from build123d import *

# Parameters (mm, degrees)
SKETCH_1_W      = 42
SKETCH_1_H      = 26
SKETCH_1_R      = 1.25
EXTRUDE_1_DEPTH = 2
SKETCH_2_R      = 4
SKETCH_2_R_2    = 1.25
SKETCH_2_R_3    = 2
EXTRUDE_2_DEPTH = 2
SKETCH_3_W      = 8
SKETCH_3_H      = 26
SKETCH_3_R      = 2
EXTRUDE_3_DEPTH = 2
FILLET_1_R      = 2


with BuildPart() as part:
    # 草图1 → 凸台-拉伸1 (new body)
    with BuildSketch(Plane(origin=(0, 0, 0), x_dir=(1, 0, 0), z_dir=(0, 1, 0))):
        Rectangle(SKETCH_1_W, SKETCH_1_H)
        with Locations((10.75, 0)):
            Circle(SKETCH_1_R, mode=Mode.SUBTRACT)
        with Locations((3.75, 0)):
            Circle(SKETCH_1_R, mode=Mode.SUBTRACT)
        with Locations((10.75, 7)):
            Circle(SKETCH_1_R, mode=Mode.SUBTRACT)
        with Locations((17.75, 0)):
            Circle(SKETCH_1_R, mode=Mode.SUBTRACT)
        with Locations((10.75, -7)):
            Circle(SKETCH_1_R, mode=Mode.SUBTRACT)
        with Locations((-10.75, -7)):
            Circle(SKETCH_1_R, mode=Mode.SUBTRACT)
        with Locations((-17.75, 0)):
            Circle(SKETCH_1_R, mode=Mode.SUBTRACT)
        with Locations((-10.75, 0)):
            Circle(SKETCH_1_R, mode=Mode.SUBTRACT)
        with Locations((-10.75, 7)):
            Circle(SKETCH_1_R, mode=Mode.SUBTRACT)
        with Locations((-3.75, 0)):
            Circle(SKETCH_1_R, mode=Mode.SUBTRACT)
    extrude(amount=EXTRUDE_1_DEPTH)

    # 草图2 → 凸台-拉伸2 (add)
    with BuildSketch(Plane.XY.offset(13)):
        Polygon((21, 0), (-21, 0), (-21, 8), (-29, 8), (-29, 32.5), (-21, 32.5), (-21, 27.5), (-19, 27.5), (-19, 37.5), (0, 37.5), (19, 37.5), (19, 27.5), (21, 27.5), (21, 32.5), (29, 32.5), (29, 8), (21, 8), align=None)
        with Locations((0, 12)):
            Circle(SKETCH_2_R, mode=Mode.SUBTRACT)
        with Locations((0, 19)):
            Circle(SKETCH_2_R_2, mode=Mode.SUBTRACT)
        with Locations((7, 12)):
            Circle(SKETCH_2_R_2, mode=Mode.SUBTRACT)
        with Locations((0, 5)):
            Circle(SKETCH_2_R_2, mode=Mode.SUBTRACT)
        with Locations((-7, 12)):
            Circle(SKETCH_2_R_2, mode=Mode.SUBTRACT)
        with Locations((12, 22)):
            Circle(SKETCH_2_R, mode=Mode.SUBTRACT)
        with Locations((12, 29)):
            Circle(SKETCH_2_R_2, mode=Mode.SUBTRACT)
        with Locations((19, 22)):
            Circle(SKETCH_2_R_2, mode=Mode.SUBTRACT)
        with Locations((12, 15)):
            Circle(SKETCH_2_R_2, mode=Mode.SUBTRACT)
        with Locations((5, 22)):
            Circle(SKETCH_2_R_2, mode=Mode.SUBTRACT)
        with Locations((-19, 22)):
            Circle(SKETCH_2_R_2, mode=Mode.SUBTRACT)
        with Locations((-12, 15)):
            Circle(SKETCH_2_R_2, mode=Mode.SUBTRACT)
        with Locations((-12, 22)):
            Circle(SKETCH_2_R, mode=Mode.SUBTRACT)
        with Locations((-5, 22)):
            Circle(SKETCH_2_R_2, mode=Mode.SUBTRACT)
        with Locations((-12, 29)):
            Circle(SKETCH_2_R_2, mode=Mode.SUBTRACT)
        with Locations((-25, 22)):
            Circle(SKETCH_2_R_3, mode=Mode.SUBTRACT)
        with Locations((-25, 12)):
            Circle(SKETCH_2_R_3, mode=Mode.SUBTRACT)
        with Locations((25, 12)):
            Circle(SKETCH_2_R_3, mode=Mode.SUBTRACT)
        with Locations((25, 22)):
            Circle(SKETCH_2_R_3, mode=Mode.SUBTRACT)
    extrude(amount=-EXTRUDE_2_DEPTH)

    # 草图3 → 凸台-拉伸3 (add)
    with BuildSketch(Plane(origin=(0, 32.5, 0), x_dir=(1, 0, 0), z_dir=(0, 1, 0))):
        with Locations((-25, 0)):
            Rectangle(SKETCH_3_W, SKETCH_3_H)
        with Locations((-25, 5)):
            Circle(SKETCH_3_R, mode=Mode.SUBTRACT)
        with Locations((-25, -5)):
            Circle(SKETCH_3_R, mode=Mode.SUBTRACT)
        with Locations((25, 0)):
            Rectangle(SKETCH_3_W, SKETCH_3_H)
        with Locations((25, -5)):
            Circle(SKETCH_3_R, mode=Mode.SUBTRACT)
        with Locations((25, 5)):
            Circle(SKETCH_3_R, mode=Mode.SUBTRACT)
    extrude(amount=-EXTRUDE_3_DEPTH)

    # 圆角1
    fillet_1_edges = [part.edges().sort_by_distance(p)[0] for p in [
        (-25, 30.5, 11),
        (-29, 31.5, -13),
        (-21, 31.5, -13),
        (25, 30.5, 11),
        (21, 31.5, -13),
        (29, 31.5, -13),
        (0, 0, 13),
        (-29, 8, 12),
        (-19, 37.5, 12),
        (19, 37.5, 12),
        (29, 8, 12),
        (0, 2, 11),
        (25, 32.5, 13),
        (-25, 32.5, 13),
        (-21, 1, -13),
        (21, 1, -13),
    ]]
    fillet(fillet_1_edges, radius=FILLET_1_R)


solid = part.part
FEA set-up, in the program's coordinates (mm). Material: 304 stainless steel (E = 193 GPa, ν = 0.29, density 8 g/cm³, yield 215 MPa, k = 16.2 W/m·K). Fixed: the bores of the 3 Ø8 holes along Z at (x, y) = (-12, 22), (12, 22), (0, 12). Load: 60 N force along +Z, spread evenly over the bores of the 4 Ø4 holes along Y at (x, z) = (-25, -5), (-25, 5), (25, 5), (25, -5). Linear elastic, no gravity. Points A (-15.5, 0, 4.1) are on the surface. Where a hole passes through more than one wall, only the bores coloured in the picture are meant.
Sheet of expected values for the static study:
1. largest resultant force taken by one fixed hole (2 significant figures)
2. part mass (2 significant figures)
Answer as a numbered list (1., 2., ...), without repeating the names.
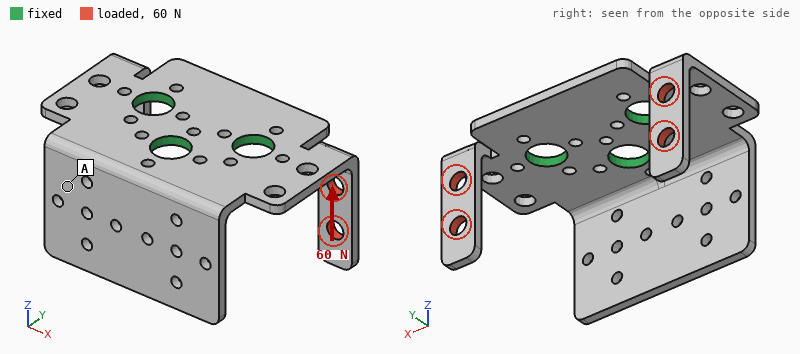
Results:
1. 34 N
2. 47 g
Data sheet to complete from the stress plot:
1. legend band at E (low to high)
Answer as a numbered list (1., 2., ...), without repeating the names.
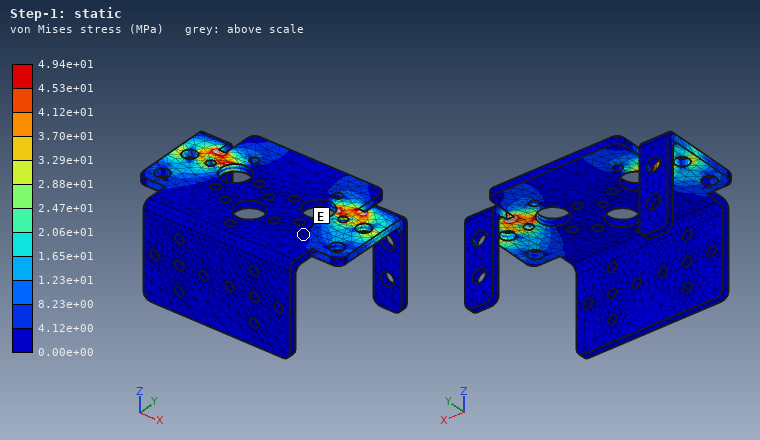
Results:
1. 0.00e+00 to 4.12e+00 MPa
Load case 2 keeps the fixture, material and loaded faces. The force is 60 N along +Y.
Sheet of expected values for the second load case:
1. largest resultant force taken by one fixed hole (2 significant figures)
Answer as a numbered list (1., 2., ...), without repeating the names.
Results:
1. 31 N
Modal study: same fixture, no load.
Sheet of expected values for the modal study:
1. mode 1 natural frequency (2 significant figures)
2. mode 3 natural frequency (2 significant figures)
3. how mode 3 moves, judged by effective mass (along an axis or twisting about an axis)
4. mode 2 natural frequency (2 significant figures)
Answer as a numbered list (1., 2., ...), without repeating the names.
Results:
1. 1600 Hz
2. 1700 Hz
3. along Y
4. 1600 Hz
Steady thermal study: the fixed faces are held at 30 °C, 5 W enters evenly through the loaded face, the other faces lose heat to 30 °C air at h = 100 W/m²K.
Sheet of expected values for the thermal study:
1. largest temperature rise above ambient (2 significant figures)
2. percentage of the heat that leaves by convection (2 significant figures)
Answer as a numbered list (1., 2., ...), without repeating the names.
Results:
1. 51 K
2. 89 %
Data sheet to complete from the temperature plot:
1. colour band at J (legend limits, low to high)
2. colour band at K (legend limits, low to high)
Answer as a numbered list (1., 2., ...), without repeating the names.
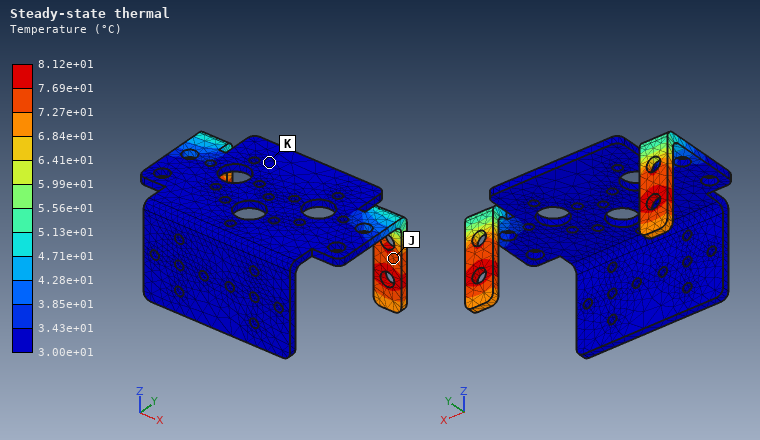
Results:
1. 7.27e+01 to 7.69e+01 °C
2. 3.00e+01 to 3.43e+01 °C
